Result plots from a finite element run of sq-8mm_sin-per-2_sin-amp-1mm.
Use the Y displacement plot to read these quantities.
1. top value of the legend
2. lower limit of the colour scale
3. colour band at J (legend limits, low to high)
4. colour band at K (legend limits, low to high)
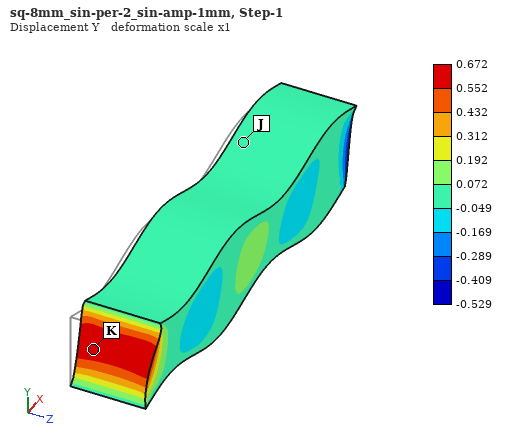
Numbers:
0.672
-0.529
-0.049 to 0.072
0.552 to 0.672
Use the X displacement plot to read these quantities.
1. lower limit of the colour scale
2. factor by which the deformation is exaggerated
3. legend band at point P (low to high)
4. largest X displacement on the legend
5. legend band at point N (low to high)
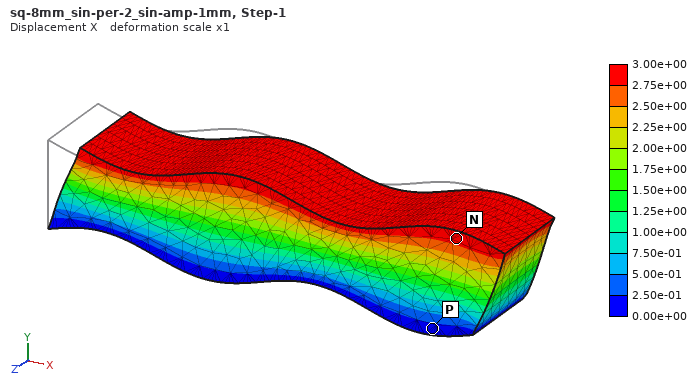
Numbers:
0.00e+00
1
0.00e+00 to 2.50e-01
3.00e+00
2.75e+00 to 3.00e+00
